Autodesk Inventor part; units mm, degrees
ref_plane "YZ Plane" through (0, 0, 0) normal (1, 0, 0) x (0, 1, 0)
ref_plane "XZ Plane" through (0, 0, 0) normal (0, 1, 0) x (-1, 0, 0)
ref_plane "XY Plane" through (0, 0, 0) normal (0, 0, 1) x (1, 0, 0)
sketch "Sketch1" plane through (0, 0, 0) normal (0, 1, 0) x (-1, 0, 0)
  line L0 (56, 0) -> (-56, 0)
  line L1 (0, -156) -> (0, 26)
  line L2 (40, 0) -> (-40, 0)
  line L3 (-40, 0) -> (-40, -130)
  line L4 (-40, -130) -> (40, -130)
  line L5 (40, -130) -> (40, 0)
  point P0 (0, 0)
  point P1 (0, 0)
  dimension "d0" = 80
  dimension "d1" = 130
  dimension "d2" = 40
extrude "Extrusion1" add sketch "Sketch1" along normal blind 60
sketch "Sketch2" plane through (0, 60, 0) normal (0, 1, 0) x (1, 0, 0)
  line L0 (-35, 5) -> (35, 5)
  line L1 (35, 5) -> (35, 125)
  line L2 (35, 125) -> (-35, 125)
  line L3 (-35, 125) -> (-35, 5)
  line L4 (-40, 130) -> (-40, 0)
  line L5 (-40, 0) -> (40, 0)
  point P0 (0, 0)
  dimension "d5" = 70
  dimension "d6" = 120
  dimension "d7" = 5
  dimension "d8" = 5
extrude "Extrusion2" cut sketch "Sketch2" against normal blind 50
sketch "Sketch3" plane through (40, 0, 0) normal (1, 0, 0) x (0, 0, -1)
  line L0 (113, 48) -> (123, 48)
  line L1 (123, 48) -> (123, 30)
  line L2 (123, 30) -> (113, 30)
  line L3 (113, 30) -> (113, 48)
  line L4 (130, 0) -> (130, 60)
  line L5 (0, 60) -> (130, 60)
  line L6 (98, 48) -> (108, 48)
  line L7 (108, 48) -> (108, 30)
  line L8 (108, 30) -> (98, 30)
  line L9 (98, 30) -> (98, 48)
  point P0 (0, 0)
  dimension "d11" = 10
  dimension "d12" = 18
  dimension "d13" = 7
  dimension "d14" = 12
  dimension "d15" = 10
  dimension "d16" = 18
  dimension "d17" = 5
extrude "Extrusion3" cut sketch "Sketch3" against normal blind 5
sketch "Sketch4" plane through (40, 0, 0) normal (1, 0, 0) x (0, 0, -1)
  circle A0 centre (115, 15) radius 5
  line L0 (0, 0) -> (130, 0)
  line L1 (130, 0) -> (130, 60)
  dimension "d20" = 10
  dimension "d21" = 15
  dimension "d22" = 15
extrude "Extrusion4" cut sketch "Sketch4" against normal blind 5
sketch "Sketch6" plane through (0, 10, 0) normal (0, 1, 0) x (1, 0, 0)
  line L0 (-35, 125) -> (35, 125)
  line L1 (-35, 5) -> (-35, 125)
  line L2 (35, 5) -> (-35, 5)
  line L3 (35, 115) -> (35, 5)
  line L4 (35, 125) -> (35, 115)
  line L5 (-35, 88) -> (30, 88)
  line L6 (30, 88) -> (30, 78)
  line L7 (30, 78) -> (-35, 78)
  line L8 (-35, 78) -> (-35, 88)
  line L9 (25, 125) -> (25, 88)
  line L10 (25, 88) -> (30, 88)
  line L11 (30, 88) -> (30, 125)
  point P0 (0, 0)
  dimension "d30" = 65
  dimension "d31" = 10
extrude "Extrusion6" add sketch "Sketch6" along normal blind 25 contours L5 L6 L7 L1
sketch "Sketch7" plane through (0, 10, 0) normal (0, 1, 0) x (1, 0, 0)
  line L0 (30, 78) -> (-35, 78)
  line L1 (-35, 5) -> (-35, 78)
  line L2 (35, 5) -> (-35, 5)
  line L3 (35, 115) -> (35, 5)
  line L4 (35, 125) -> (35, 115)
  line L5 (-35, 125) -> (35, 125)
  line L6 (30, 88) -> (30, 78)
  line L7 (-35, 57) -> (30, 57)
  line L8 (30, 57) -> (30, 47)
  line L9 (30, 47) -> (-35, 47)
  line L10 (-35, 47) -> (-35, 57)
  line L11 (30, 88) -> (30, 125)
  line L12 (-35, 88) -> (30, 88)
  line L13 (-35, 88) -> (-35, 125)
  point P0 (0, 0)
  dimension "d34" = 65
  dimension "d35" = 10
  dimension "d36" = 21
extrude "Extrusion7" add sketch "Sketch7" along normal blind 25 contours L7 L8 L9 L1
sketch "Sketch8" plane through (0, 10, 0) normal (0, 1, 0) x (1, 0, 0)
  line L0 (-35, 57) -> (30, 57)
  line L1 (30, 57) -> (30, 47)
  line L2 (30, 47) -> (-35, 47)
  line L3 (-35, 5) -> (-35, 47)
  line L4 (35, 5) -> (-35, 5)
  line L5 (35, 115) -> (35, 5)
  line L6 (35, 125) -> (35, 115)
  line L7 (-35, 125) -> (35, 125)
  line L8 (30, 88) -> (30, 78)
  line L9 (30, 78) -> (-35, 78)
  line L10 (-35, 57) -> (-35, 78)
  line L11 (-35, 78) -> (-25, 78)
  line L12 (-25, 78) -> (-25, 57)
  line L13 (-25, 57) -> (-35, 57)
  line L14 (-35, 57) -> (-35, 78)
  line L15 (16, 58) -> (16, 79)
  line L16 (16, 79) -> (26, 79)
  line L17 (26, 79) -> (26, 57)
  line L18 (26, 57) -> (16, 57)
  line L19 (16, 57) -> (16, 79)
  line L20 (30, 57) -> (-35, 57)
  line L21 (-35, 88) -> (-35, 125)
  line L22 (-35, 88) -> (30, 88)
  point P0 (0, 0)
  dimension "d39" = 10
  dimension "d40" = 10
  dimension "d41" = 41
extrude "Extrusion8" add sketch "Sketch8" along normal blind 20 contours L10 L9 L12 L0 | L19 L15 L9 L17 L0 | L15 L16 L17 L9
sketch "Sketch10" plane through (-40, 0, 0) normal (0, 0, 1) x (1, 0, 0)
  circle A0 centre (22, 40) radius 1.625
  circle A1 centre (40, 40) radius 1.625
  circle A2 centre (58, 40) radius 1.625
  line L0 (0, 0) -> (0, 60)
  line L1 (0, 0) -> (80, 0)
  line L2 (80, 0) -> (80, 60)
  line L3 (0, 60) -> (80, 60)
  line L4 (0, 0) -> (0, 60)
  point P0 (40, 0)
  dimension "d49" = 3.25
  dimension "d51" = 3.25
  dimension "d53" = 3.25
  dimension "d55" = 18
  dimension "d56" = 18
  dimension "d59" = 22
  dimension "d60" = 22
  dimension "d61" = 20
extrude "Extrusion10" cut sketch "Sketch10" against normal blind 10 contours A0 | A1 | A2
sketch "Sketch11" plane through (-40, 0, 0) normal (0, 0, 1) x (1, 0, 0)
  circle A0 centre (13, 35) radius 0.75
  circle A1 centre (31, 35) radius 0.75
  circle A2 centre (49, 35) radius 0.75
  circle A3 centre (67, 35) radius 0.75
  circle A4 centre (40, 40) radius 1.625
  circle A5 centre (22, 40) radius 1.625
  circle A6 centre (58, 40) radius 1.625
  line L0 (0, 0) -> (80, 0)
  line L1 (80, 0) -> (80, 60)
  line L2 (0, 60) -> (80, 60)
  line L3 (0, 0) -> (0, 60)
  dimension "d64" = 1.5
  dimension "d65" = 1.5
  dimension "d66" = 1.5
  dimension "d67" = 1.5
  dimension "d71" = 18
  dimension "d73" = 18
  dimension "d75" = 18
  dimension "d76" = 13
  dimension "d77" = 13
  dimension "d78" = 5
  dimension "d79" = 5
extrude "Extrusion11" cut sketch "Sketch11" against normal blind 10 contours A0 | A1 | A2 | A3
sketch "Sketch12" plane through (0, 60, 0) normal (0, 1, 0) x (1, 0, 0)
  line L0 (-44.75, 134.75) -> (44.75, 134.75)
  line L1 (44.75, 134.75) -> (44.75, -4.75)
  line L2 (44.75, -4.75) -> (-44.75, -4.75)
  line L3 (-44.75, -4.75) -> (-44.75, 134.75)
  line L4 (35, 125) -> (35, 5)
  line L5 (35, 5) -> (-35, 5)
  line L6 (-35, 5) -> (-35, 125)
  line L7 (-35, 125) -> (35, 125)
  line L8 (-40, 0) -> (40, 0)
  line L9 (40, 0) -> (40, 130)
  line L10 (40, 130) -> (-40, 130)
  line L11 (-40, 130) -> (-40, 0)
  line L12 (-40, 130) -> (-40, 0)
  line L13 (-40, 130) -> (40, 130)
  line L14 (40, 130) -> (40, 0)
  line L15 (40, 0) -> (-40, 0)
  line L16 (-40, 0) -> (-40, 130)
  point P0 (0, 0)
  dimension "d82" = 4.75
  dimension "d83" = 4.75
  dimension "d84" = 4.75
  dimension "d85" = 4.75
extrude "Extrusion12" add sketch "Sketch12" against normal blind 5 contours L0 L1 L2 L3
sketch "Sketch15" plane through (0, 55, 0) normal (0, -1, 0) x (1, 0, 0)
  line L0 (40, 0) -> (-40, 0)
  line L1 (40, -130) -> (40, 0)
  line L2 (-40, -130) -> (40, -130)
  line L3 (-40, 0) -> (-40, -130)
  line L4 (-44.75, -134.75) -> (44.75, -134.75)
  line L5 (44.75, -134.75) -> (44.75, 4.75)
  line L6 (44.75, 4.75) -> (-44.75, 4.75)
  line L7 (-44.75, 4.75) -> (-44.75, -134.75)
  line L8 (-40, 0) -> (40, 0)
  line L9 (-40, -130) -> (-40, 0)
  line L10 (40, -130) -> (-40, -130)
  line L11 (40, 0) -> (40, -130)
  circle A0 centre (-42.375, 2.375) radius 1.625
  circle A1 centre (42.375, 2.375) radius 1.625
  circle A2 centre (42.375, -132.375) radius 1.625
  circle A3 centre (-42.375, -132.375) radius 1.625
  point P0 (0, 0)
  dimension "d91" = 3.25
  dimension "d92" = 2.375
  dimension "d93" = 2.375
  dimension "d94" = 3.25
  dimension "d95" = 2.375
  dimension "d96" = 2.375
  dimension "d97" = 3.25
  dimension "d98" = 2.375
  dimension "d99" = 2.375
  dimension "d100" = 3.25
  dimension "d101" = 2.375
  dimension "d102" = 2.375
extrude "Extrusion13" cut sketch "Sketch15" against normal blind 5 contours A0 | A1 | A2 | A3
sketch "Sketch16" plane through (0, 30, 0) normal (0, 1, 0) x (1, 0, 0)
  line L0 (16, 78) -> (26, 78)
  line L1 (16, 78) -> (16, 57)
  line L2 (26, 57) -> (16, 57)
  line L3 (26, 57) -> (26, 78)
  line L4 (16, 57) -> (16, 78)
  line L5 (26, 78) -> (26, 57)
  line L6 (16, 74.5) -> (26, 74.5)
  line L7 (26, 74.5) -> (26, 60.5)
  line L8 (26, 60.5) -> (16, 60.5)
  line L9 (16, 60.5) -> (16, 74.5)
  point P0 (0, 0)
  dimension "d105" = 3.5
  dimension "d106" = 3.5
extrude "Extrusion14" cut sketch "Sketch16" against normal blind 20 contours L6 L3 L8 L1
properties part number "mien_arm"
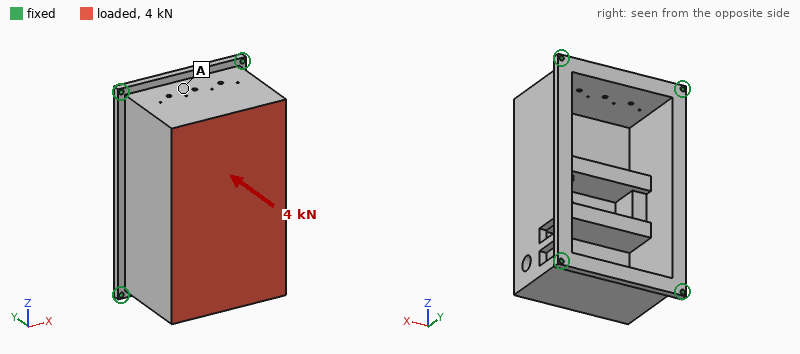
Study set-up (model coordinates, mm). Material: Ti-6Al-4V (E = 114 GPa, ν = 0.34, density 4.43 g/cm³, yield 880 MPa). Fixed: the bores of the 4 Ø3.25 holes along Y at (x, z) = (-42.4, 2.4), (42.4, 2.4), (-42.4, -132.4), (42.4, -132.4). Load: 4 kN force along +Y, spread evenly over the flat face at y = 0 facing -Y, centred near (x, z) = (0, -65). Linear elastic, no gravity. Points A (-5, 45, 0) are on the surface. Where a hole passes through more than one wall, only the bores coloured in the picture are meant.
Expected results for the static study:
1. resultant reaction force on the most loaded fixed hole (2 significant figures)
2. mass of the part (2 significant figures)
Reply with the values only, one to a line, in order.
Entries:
1.3 kN
1.1 kg
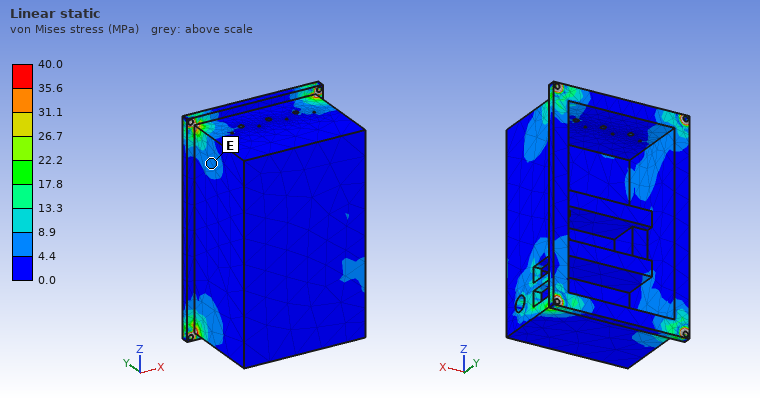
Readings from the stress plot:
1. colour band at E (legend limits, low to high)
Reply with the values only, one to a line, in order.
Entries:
4.4 to 8.9 MPa
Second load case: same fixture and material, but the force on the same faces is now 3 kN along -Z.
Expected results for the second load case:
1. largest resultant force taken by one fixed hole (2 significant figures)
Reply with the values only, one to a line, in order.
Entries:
1.2 kN
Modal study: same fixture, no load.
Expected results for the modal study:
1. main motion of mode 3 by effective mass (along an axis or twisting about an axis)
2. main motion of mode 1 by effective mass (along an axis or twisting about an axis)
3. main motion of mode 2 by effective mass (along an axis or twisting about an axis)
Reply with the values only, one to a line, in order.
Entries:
along Y
along X
along Y
